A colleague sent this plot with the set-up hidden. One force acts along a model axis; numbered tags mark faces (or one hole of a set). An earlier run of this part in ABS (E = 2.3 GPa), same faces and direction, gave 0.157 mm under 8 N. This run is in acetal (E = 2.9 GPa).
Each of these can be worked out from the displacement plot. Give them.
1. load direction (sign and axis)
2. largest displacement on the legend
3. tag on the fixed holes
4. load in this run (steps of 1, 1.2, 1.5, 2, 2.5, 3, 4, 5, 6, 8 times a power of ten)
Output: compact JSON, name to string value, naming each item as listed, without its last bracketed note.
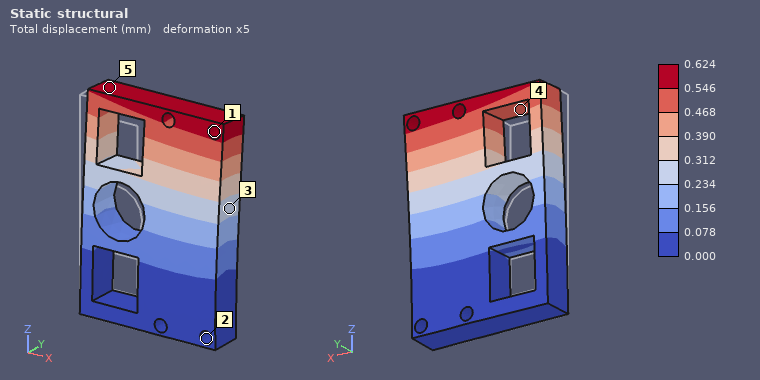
{"load direction": "+Y", "largest displacement on the legend": "0.624 mm", "tag on the fixed holes": "2", "load in this run": "40 N"}
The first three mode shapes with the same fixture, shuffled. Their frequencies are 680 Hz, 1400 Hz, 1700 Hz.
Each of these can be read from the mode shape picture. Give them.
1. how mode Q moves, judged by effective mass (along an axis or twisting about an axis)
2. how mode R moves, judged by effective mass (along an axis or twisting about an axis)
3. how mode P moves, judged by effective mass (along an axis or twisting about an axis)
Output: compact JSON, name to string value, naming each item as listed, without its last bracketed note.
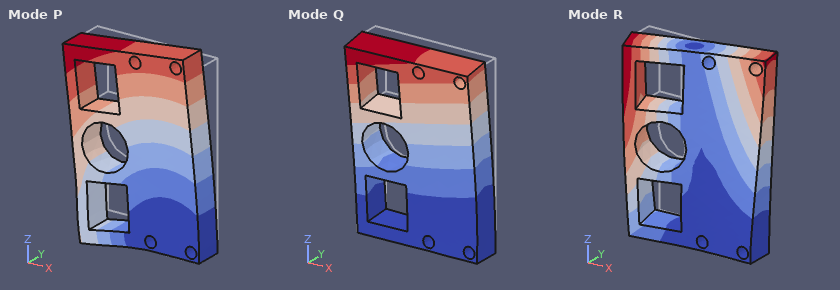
{"how mode Q moves, judged by effective mass": "along Y", "how mode R moves, judged by effective mass": "twisting about Z", "how mode P moves, judged by effective mass": "along X"}
